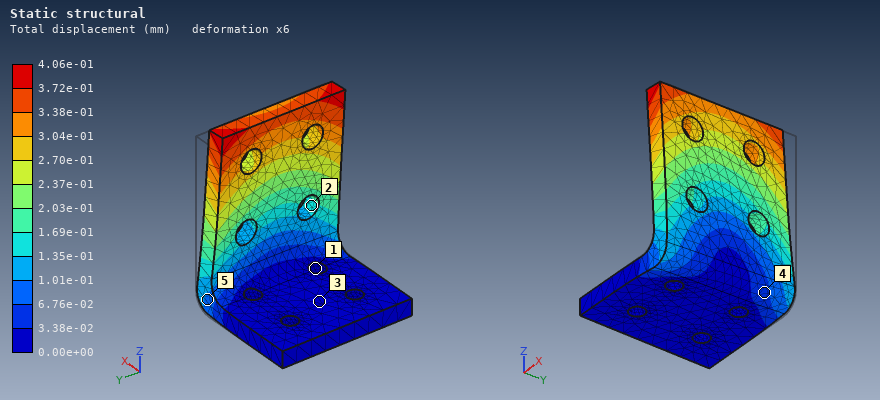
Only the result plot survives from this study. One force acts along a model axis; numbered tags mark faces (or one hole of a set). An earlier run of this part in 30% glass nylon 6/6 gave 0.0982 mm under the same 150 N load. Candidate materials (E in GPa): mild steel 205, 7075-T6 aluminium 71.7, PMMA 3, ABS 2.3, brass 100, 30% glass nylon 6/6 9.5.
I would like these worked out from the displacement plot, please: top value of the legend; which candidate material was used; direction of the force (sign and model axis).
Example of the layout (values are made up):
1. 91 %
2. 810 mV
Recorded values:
1. 4.06e-01 mm
2. ABS
3. -Y
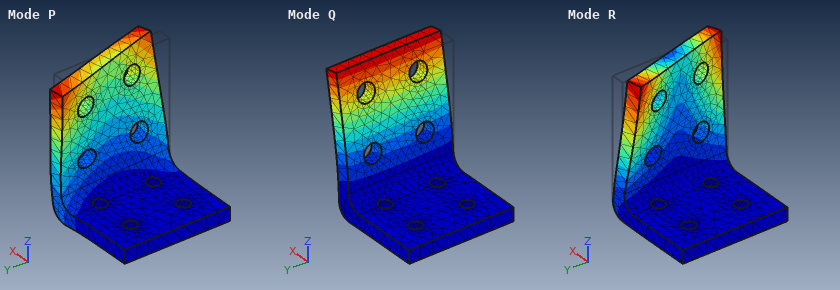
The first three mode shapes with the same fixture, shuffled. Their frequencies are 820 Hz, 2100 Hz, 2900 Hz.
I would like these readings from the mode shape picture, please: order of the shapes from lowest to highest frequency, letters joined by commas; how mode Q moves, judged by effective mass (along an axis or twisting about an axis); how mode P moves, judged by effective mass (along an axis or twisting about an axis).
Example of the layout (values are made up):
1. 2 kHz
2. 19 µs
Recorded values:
1. Q, R, P
2. along X
3. along Y
